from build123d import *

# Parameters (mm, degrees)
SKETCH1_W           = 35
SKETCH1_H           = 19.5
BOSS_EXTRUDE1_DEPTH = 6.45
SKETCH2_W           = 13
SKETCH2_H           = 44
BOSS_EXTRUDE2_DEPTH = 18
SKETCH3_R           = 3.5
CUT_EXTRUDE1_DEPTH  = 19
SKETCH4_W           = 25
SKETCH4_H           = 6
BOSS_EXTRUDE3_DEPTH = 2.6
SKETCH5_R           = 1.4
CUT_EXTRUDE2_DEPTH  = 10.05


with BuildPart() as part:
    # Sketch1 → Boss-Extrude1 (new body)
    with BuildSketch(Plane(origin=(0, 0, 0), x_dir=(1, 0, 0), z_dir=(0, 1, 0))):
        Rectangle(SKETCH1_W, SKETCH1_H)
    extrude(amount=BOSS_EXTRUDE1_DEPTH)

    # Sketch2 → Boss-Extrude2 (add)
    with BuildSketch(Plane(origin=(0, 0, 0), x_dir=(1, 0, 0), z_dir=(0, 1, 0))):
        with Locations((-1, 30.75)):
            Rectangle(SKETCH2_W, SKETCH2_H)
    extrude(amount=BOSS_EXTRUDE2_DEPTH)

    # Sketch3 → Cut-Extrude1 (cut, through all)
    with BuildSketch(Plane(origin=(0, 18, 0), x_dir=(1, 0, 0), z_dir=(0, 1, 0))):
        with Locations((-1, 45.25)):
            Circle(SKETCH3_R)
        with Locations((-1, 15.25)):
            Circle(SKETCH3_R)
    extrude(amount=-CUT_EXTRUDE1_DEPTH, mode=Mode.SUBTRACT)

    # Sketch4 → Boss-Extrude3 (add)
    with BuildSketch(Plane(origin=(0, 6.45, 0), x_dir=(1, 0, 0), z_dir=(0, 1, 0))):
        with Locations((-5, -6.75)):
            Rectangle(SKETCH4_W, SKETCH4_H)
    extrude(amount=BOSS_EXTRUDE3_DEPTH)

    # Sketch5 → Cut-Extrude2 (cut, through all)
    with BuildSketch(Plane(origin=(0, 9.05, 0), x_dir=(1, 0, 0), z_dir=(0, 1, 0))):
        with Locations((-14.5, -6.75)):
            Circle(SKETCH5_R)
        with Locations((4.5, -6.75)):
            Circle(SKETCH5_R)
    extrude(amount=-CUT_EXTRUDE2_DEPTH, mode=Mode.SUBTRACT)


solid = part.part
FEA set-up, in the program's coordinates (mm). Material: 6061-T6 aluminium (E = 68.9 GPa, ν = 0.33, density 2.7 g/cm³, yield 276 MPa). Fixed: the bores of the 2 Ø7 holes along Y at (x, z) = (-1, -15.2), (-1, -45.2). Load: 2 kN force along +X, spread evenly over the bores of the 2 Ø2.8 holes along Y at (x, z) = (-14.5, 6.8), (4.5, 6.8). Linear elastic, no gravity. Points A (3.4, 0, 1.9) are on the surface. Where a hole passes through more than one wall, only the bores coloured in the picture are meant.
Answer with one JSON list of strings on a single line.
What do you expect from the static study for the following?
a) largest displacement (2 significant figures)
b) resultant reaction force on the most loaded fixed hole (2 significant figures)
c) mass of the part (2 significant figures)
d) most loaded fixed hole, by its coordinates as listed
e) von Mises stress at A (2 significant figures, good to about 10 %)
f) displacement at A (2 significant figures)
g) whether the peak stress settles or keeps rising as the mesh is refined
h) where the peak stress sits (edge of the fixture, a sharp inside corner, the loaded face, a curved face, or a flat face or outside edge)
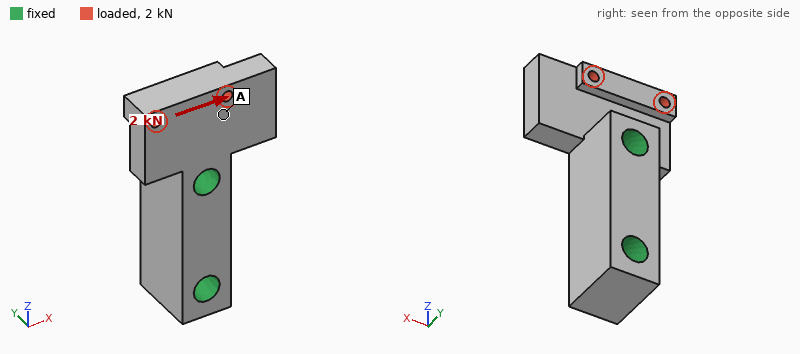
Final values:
["0.12 mm", "2.2 kN", "36 g", "(-1, -15.2)", "24 MPa", "0.056 mm", "keeps rising", "a sharp inside corner"]
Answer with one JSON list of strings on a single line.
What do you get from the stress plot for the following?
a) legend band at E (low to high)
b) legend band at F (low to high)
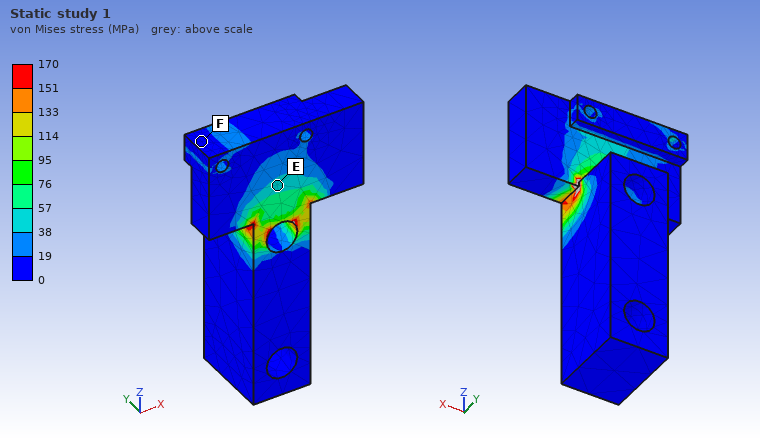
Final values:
["38 to 57 MPa", "0 to 19 MPa"]
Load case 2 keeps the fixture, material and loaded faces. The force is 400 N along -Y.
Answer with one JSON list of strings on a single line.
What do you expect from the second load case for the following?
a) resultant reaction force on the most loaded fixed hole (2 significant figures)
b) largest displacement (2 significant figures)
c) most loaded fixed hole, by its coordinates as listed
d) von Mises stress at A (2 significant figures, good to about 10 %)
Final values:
["410 N", "52 µm", "(-1, -15.2)", "11 MPa"]
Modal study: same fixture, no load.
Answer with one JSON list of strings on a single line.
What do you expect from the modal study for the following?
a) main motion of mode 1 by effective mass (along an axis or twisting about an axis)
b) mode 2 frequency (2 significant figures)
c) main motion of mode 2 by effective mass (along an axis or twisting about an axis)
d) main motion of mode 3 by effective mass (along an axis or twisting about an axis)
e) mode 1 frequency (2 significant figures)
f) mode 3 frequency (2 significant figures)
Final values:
["along Y", "8100 Hz", "along X", "twisting about Z", "7100 Hz", "9400 Hz"]
